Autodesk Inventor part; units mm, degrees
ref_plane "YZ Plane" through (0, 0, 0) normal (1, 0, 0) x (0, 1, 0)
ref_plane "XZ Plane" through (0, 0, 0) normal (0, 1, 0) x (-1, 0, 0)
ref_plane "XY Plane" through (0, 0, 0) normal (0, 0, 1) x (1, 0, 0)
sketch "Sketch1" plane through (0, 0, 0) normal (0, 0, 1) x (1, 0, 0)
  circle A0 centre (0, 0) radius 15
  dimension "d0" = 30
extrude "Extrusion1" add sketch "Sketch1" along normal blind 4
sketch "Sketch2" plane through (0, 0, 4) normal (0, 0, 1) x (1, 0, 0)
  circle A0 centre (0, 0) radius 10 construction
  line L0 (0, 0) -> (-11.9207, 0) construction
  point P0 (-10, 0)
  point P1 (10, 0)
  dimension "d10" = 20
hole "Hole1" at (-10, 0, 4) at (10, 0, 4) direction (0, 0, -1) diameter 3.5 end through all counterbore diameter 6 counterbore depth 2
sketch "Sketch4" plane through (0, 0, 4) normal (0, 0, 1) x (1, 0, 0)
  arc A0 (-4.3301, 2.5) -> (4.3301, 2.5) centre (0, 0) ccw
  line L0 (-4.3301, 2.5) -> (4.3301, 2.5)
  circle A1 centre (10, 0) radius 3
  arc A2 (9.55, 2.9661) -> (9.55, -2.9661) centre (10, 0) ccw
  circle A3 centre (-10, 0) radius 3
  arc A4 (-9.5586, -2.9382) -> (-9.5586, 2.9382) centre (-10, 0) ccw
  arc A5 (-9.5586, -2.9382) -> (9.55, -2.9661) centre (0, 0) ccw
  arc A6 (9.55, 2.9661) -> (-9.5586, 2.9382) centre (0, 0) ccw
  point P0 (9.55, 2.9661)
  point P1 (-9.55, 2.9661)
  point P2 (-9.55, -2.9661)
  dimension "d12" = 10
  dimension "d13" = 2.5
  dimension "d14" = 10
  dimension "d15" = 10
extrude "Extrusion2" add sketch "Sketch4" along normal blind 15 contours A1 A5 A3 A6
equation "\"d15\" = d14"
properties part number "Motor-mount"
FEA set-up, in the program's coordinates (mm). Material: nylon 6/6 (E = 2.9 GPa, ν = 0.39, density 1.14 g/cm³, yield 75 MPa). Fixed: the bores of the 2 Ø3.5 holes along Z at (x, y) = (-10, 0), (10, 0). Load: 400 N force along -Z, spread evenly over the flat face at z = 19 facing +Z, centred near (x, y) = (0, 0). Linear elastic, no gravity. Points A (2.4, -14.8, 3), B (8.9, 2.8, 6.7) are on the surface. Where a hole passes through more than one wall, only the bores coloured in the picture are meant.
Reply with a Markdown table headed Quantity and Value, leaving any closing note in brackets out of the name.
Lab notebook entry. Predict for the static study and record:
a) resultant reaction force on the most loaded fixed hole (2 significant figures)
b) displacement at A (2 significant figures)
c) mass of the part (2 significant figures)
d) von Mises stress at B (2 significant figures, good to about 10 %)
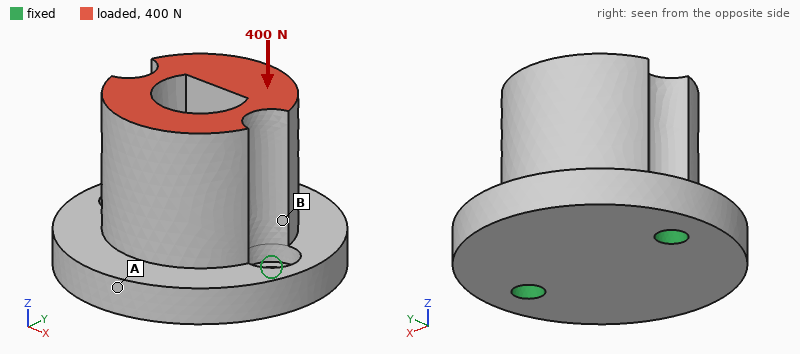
| Quantity | Value |
|---|---|
| resultant reaction force on the most loaded fixed hole | 210 N |
| displacement at A | 34 µm |
| mass of the part | 6.9 g |
| von Mises stress at B | 5.3 MPa |
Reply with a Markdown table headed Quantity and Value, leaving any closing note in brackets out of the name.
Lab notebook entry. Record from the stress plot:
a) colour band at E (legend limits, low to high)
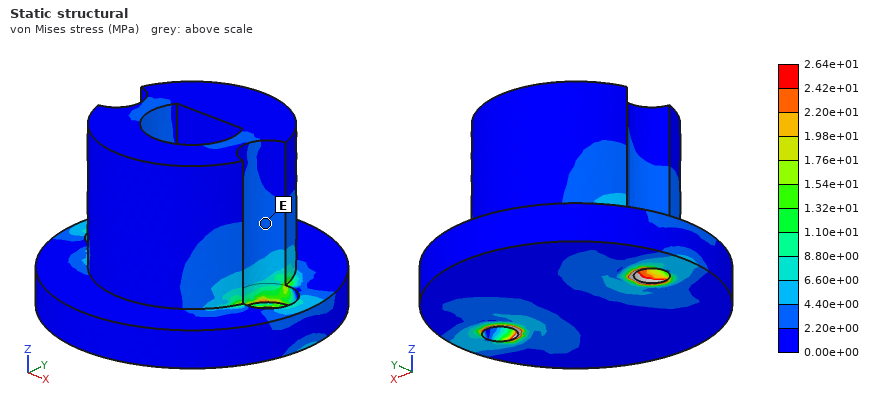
| Quantity | Value |
|---|---|
| colour band at E | 2.20e+00 to 4.40e+00 MPa |
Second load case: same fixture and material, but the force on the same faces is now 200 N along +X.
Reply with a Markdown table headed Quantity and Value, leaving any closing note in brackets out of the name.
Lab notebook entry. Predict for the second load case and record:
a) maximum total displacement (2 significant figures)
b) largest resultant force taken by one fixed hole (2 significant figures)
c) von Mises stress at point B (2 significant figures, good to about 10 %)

| Quantity | Value |
|---|---|
| maximum total displacement | 0.11 mm |
| largest resultant force taken by one fixed hole | 210 N |
| von Mises stress at point B | 5.7 MPa |
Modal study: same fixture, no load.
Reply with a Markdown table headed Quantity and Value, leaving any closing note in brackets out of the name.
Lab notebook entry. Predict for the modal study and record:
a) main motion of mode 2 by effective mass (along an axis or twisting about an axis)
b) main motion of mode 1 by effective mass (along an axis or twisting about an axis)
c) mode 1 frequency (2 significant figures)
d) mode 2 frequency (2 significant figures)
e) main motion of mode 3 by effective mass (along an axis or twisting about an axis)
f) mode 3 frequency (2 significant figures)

| Quantity | Value |
|---|---|
| main motion of mode 2 by effective mass | along X |
| main motion of mode 1 by effective mass | along Y |
| mode 1 frequency | 1600 Hz |
| mode 2 frequency | 5500 Hz |
| main motion of mode 3 by effective mass | along Z |
| mode 3 frequency | 6200 Hz |
